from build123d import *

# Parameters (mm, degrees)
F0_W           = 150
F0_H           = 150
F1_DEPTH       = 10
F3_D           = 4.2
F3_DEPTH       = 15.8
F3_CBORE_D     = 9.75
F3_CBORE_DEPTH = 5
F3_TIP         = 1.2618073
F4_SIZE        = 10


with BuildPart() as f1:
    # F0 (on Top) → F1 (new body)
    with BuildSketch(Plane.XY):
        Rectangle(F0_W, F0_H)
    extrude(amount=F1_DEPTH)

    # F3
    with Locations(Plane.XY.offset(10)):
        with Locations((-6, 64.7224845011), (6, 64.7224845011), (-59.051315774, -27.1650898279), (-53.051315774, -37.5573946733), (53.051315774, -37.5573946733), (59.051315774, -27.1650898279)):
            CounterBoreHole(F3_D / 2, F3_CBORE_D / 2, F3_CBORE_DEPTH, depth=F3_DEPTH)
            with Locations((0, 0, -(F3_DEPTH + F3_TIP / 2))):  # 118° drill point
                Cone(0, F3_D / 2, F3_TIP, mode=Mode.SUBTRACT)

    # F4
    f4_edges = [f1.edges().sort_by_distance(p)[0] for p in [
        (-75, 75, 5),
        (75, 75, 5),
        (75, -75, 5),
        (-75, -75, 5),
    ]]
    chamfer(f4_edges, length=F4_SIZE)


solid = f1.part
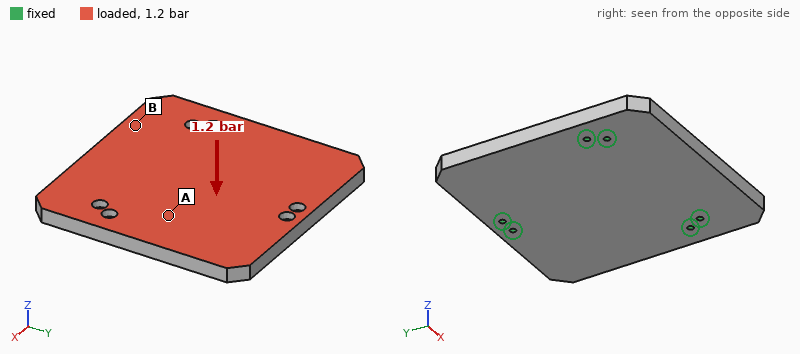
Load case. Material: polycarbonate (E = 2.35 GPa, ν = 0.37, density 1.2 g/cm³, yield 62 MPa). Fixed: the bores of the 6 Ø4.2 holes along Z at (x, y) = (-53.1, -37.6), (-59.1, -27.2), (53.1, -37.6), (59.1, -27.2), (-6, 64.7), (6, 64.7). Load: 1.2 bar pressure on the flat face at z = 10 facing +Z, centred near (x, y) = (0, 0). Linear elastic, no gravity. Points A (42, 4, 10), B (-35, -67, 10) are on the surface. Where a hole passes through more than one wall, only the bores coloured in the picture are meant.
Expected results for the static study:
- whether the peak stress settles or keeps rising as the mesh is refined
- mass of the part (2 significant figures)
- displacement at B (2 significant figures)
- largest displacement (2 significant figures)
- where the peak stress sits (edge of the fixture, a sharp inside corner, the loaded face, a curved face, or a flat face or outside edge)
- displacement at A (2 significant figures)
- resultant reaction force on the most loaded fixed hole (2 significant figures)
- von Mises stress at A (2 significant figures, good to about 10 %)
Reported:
keeps rising
260 g
0.39 mm
1.2 mm
edge of the fixture
0.47 mm
620 N
6.2 MPa
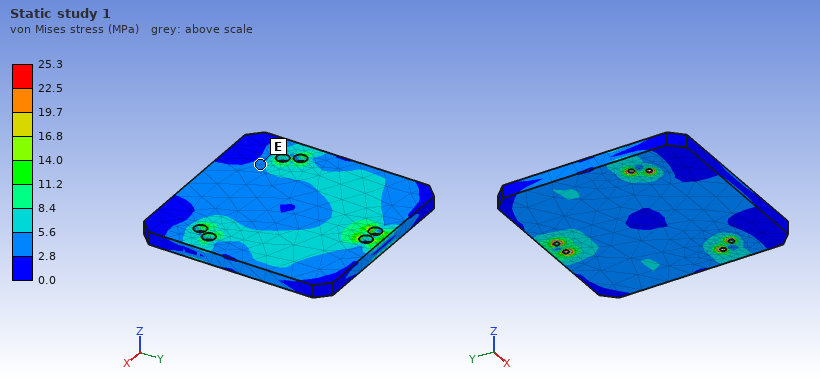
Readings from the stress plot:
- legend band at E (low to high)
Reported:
2.8 to 5.6 MPa
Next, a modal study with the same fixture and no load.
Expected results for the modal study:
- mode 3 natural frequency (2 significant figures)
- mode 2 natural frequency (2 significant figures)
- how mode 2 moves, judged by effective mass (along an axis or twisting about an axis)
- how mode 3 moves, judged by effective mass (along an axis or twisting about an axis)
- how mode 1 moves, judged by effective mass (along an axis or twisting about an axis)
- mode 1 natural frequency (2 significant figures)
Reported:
730 Hz
570 Hz
along Z
along Z
twisting about Y
510 Hz
